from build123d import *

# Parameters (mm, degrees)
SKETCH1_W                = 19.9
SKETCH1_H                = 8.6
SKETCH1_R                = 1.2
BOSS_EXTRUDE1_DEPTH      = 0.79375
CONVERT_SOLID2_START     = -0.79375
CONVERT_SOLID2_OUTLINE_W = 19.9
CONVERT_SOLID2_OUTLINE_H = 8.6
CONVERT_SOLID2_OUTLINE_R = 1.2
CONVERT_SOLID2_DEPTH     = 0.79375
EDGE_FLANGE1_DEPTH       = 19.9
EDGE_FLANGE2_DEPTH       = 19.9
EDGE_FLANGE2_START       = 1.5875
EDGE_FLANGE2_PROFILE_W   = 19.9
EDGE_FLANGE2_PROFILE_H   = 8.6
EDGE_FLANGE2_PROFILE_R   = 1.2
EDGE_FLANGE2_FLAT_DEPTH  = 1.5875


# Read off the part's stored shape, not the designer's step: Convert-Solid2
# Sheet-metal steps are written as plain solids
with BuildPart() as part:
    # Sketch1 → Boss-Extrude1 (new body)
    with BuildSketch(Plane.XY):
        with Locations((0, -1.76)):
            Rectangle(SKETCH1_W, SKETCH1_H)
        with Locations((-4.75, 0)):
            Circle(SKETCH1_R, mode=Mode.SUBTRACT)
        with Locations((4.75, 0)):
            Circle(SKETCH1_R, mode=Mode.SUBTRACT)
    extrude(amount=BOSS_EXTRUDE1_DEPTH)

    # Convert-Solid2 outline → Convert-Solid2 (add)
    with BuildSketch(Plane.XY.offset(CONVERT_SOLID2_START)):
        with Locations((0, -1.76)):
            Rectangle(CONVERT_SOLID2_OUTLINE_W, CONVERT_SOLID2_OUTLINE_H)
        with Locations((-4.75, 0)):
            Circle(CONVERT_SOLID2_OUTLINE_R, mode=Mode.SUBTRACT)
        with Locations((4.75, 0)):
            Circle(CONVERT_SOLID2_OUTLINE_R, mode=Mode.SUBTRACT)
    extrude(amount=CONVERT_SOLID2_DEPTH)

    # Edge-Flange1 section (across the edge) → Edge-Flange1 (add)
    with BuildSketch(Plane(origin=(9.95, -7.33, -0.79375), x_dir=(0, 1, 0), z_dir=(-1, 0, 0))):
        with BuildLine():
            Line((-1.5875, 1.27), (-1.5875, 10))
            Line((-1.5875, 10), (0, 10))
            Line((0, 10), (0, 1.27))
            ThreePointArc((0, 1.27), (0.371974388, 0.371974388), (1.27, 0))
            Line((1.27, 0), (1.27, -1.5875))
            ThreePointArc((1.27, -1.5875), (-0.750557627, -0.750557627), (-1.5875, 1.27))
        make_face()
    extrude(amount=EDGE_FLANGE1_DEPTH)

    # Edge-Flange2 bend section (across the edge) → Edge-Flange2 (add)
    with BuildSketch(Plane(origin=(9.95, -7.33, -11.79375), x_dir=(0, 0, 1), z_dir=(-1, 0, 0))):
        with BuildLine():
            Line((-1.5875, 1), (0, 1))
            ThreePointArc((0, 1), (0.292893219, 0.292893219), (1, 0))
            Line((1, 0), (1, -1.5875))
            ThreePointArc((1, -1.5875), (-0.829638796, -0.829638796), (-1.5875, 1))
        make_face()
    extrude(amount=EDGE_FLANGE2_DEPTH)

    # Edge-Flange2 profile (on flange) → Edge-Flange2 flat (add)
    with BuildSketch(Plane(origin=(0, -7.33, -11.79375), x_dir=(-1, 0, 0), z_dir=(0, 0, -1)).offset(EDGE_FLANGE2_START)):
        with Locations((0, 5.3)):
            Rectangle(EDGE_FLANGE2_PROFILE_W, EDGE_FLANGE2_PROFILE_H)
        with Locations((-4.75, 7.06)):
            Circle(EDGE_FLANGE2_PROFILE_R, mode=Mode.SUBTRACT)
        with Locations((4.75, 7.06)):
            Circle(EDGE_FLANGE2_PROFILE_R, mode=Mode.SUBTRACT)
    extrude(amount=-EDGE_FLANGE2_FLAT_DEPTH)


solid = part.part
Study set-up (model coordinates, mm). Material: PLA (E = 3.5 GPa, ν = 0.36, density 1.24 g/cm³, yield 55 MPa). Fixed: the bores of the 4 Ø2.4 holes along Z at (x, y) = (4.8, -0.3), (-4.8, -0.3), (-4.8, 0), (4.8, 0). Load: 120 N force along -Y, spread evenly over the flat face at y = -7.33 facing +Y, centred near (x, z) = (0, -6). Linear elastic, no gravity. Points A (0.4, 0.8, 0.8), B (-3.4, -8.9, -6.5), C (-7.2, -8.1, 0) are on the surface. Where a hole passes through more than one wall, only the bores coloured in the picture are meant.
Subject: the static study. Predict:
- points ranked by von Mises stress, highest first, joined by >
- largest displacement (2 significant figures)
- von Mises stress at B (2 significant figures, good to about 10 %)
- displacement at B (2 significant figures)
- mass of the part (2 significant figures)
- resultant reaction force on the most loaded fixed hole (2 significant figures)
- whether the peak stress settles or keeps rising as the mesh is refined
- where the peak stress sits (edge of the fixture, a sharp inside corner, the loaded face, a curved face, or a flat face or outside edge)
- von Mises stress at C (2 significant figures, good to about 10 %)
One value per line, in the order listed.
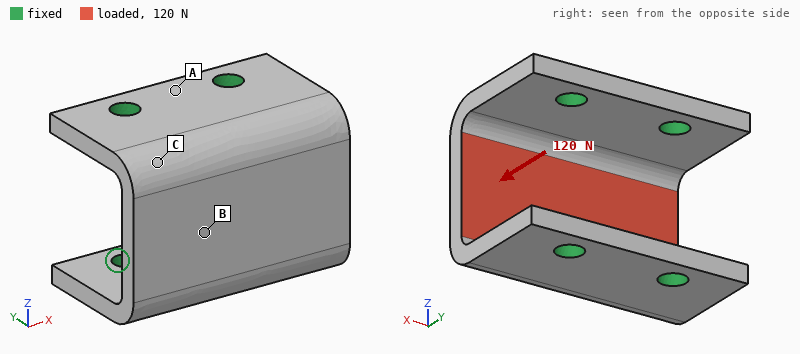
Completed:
B > C > A
71 µm
12 MPa
57 µm
1.2 g
33 N
keeps rising
edge of the fixture
5.8 MPa
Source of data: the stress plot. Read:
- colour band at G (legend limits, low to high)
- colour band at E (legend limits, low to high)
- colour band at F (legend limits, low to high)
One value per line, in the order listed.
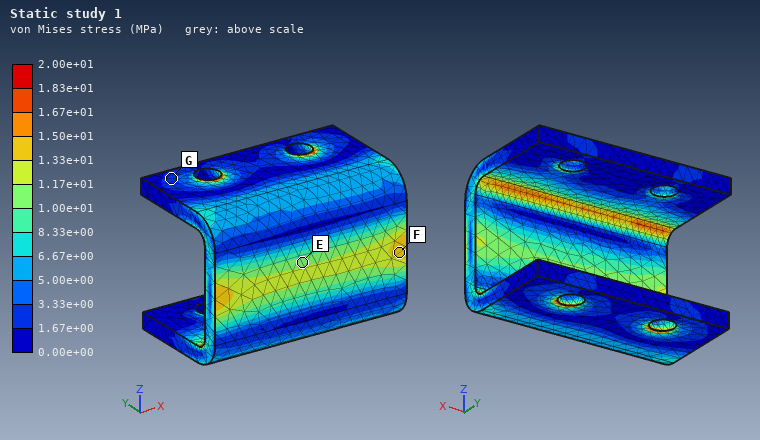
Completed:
1.67e+00 to 3.33e+00 MPa
1.00e+01 to 1.17e+01 MPa
1.33e+01 to 1.50e+01 MPa
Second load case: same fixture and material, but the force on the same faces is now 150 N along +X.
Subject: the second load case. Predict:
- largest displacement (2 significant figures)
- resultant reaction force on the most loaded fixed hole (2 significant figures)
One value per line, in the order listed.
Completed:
35 µm
58 N
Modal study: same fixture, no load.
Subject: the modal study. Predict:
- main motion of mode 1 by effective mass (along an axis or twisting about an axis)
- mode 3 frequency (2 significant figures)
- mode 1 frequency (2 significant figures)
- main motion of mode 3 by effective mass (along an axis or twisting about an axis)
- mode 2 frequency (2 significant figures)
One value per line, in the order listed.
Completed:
along Z
12 kHz
5800 Hz
twisting about Y
12 kHz
